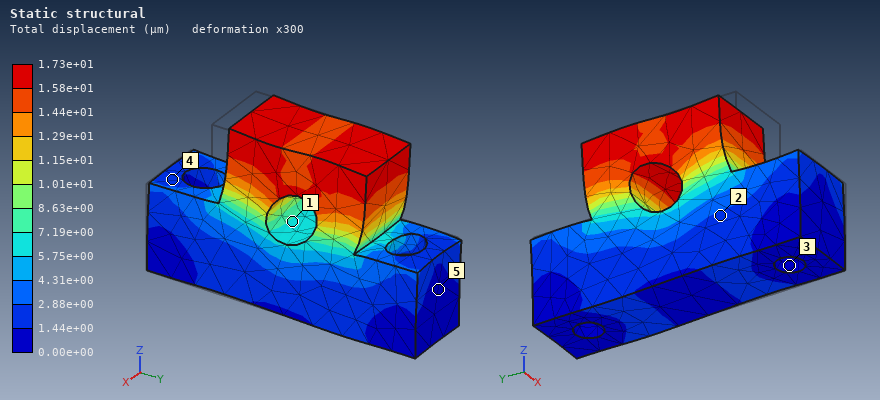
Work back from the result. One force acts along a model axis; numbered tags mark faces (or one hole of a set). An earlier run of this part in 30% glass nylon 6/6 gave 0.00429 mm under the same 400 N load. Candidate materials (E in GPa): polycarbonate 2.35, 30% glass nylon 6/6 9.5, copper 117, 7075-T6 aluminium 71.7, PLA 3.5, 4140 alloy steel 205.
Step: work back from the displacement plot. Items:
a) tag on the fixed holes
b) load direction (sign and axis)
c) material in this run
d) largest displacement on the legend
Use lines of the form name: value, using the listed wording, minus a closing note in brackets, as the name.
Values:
tag on the fixed holes: 3
load direction: +Y
material in this run: polycarbonate
largest displacement on the legend: 1.73e+01 µm
